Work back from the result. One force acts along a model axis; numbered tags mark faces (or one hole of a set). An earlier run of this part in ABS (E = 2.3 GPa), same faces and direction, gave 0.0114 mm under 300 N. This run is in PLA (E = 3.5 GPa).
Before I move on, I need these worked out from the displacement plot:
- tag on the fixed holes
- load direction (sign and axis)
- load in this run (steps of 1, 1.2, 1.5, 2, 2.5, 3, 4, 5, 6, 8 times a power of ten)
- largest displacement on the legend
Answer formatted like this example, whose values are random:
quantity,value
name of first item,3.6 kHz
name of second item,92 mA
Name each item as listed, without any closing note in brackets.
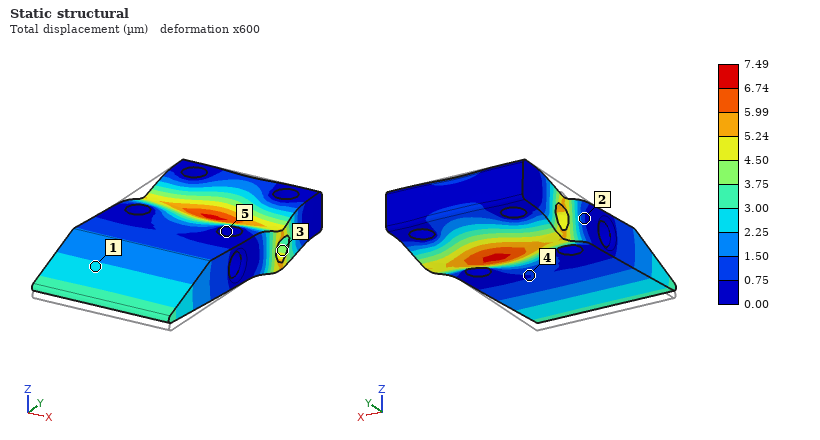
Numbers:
quantity,value
tag on the fixed holes,5
load direction,-Z
load in this run,300 N
largest displacement on the legend,7.49 µm
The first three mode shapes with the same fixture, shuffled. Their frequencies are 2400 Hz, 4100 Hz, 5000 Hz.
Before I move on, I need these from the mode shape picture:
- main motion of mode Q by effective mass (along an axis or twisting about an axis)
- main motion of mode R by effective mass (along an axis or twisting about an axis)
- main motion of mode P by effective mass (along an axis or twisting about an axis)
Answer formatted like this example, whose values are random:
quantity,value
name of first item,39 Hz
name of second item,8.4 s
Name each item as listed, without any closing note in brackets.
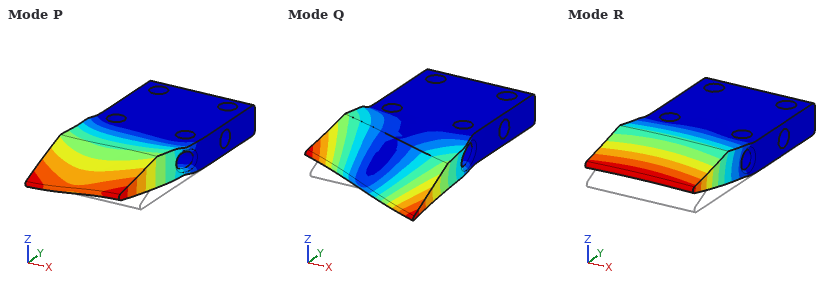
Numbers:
quantity,value
main motion of mode Q by effective mass,twisting about Y
main motion of mode R by effective mass,along Z
main motion of mode P by effective mass,along X
